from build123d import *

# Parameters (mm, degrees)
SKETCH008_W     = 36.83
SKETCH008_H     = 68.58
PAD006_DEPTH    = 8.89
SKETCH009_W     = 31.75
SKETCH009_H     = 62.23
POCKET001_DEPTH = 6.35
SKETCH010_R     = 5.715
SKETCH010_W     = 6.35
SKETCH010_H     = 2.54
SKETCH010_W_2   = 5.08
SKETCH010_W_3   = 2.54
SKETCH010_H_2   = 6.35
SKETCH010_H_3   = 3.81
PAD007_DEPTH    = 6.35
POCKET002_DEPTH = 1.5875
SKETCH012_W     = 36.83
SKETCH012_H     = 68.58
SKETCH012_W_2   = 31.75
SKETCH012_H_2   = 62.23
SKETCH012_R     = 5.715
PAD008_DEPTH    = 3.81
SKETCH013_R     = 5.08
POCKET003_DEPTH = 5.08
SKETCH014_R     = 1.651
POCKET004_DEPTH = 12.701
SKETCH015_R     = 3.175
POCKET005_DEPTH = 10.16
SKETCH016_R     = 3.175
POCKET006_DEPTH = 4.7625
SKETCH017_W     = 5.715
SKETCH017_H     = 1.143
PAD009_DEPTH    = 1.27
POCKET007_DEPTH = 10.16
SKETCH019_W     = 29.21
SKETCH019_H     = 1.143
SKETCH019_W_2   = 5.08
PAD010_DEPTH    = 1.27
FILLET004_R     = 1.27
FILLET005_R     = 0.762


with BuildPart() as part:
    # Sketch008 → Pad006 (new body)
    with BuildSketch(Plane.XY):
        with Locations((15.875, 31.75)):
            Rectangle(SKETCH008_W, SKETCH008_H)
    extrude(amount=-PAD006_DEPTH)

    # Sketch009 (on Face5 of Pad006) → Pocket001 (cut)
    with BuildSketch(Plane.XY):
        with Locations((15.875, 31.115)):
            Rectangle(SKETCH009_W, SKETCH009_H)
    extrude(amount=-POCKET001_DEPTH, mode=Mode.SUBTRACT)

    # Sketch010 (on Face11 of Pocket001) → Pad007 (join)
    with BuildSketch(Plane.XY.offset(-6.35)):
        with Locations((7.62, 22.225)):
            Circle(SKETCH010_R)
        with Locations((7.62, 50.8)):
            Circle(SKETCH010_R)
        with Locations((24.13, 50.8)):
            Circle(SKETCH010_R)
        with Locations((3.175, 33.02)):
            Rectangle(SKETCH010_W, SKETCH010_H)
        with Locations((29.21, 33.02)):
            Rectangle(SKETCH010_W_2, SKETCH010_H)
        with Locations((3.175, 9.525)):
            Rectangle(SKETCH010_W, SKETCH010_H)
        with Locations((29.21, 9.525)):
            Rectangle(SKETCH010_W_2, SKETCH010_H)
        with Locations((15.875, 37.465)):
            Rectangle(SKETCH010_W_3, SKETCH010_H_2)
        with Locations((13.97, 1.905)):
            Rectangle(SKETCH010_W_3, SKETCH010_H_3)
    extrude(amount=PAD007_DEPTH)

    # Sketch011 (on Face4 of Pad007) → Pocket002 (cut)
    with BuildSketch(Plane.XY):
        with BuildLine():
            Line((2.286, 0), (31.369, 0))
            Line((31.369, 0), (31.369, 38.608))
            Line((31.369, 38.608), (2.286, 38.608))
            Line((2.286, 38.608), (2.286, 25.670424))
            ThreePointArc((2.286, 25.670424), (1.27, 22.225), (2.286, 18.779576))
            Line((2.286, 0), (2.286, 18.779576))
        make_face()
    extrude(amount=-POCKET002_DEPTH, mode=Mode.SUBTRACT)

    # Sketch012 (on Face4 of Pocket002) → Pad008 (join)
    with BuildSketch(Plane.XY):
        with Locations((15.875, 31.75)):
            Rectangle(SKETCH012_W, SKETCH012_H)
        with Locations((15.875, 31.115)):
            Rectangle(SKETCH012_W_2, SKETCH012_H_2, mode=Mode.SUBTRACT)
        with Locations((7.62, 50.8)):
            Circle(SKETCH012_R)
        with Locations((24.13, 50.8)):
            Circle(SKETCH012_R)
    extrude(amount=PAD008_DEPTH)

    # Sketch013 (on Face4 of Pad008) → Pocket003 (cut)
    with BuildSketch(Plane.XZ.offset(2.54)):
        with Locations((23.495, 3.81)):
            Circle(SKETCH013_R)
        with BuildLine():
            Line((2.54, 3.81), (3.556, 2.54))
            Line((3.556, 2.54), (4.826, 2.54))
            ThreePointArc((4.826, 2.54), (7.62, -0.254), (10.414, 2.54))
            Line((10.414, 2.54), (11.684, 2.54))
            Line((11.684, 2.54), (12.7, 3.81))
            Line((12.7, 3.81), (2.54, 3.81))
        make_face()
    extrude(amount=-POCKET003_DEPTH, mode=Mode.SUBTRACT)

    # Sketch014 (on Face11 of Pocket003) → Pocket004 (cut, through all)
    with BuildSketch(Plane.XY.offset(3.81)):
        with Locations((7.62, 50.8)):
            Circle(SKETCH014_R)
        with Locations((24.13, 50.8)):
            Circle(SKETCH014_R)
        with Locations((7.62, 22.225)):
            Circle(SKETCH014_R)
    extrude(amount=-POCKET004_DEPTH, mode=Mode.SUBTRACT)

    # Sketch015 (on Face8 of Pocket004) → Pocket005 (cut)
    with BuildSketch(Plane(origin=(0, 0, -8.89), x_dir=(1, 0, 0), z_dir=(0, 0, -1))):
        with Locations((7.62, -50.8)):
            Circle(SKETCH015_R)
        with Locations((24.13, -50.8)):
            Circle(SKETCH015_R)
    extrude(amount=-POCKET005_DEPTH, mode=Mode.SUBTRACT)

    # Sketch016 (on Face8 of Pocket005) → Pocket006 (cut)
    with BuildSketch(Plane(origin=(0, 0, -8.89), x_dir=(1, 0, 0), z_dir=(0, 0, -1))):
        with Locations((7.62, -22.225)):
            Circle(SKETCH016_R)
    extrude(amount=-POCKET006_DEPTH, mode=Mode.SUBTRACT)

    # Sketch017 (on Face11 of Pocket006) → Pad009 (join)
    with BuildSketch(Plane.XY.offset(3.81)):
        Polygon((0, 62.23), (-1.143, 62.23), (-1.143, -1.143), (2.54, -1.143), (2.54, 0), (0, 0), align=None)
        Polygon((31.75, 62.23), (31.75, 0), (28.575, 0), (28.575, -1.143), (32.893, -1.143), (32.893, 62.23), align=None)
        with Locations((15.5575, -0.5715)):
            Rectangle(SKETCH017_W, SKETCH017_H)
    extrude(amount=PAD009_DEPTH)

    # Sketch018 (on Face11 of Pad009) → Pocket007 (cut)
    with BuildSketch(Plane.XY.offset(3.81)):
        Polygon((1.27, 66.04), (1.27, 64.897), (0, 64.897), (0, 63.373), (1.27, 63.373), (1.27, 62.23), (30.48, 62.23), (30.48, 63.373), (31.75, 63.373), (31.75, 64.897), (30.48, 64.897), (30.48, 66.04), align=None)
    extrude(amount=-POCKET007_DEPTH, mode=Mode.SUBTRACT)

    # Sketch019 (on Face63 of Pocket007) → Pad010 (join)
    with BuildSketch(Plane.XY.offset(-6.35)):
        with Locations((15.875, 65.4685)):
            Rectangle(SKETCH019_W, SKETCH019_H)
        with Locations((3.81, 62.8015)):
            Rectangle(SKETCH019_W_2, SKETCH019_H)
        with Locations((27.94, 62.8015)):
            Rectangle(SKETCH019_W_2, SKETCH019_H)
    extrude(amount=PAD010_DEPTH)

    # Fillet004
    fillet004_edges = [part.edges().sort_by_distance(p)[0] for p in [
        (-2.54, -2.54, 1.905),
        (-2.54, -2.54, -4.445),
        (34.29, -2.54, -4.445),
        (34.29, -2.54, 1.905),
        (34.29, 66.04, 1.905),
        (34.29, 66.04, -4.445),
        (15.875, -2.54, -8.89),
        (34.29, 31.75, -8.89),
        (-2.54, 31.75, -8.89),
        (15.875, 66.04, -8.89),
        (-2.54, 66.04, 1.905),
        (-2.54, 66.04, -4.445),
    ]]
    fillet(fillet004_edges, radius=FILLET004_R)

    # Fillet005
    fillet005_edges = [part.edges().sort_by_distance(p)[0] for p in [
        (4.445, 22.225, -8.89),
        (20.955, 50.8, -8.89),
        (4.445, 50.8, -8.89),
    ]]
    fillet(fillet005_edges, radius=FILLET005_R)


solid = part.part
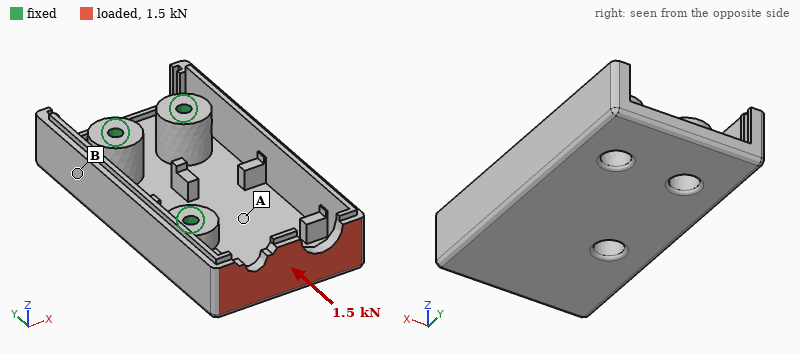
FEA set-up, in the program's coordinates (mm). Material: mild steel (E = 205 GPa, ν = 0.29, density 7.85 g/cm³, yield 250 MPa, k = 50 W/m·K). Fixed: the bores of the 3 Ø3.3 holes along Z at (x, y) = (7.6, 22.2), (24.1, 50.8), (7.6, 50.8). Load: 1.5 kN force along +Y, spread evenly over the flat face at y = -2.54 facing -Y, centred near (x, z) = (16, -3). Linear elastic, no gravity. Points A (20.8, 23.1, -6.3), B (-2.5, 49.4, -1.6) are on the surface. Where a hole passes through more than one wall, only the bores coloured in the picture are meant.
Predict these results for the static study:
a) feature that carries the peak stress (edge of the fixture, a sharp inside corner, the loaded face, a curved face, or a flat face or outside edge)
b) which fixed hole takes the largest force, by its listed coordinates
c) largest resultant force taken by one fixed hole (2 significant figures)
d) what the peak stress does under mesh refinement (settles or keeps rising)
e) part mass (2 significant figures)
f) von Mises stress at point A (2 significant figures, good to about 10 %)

edge of the fixture
(7.6, 22.2)
950 N
keeps rising
100 g
20 MPa
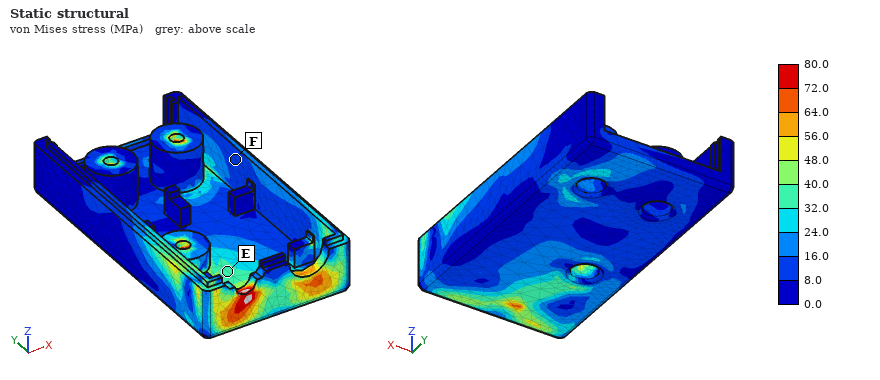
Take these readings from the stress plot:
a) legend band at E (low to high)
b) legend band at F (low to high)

32.0 to 40.0 MPa
8.0 to 16.0 MPa
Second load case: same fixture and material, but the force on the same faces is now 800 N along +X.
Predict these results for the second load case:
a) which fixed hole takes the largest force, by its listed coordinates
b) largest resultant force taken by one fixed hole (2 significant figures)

(7.6, 22.2)
1.3 kN
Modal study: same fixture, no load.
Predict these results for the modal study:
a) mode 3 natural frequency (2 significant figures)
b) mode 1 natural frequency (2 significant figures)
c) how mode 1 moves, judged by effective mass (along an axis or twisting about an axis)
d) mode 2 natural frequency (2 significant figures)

6200 Hz
2300 Hz
along Z
5600 Hz
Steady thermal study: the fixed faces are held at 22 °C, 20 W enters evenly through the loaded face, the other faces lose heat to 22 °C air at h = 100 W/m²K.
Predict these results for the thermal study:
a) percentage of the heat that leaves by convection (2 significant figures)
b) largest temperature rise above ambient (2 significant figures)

72 %
67 K
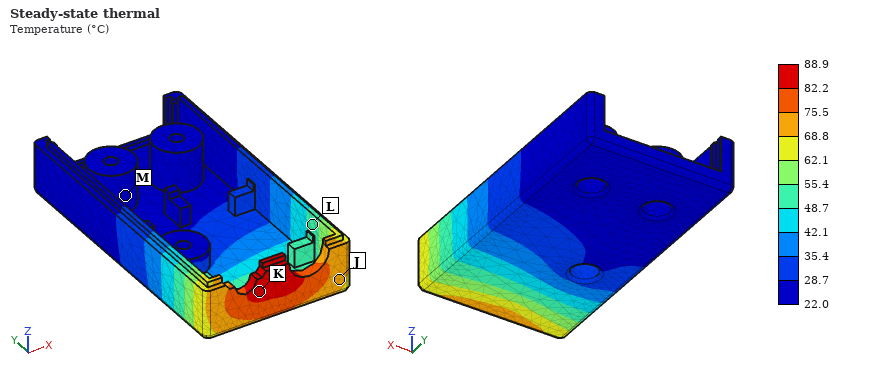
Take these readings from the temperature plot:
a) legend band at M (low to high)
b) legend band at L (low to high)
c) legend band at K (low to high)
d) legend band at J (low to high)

22.0 to 28.7 °C
48.7 to 55.4 °C
82.2 to 88.9 °C
68.8 to 75.5 °C
